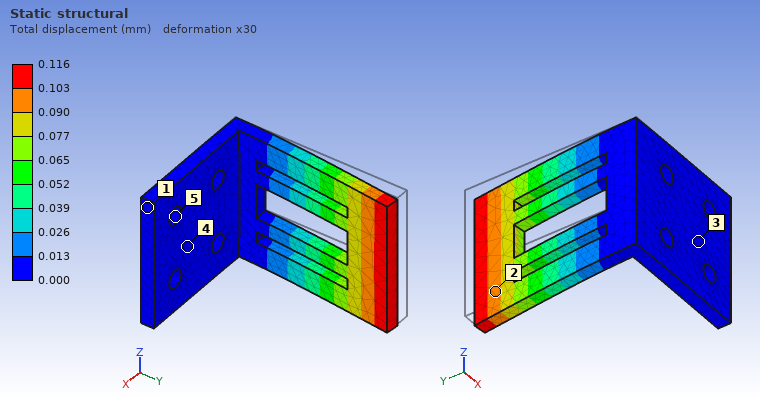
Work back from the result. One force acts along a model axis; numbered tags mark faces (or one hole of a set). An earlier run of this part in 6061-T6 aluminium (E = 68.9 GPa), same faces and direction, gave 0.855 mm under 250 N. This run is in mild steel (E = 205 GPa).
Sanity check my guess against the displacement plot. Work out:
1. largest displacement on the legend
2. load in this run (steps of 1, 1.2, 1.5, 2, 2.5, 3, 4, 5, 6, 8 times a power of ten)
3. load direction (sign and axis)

0.116 mm
100 N
+X
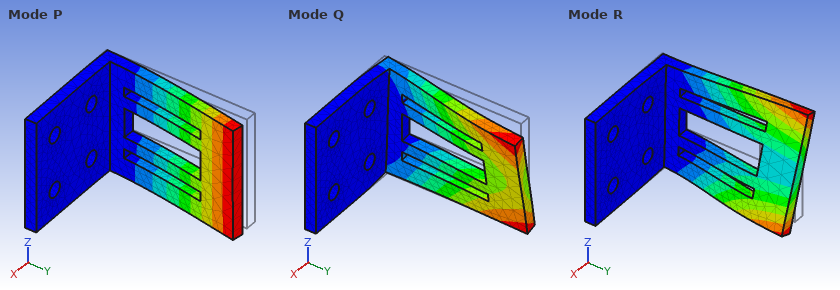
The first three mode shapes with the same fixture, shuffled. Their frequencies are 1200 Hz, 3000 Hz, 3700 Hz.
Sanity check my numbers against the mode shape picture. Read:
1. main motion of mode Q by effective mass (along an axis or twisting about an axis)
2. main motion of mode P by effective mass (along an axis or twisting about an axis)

along Z
along X
